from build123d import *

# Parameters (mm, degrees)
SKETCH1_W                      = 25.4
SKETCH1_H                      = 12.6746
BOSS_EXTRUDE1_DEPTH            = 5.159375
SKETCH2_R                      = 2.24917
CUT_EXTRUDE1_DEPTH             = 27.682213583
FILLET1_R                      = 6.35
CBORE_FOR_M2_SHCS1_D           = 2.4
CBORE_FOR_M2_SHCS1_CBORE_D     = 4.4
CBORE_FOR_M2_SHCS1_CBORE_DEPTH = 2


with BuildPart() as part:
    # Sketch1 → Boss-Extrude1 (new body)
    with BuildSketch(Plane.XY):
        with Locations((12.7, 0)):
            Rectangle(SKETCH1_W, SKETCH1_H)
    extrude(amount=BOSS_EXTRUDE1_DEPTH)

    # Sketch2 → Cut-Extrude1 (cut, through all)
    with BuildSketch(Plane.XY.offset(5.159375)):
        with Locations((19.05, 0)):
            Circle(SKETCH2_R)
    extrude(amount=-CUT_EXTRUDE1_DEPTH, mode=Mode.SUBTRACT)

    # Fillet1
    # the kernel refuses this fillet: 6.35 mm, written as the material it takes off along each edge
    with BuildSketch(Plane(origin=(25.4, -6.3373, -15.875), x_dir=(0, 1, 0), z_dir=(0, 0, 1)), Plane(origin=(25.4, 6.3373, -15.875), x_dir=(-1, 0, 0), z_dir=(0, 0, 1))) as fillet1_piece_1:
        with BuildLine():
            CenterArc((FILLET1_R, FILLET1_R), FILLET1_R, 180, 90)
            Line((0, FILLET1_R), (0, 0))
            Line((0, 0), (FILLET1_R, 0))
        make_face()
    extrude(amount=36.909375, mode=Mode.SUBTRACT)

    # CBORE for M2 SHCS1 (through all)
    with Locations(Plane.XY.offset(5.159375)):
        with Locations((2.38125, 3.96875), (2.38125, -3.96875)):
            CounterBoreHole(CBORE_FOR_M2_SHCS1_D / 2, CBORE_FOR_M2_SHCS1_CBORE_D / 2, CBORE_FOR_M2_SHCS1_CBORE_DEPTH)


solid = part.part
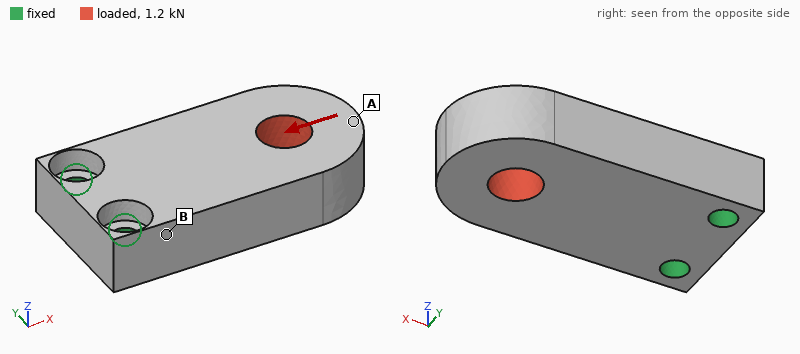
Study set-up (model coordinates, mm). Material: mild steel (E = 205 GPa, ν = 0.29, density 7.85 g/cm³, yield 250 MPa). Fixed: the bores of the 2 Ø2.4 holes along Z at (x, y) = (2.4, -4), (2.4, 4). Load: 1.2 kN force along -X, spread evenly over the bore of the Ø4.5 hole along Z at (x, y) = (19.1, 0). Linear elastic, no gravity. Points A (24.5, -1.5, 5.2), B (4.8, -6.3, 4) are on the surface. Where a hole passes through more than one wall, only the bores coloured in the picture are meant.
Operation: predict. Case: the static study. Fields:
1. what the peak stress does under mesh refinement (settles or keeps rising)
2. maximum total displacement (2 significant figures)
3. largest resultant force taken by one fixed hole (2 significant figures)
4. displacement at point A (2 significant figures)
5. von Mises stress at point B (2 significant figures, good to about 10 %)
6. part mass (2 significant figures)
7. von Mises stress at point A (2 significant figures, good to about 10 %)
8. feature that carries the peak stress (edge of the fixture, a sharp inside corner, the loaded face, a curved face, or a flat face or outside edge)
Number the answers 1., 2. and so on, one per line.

1. keeps rising
2. 7.1 µm
3. 600 N
4. 6.8 µm
5. 27 MPa
6. 11 g
7. 14 MPa
8. edge of the fixture
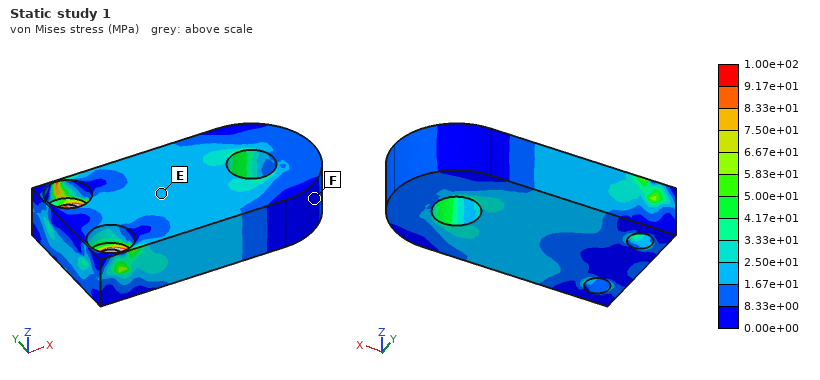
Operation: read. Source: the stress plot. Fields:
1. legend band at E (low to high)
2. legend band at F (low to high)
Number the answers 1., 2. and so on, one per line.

1. 1.67e+01 to 2.50e+01 MPa
2. 0.00e+00 to 8.33e+00 MPa
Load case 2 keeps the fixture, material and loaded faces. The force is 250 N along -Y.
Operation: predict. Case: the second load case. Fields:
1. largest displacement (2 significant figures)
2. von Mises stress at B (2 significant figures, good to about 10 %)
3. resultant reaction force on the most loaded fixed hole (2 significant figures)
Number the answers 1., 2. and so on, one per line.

1. 5.5 µm
2. 20 MPa
3. 460 N
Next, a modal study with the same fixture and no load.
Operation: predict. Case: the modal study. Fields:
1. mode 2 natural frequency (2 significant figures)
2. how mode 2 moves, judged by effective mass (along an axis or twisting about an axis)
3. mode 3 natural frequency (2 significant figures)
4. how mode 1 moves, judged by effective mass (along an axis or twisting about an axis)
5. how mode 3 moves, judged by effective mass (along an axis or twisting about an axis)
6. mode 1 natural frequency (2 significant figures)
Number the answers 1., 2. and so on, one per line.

1. 17 kHz
2. along Y
3. 26 kHz
4. along Z
5. twisting about X
6. 6900 Hz
